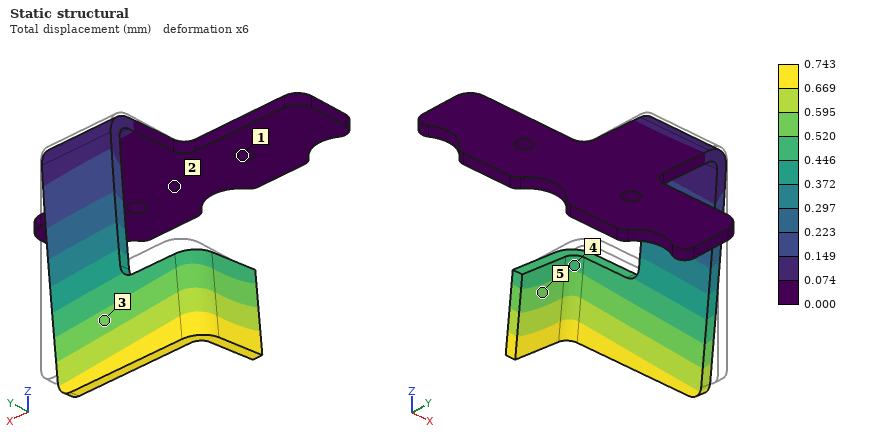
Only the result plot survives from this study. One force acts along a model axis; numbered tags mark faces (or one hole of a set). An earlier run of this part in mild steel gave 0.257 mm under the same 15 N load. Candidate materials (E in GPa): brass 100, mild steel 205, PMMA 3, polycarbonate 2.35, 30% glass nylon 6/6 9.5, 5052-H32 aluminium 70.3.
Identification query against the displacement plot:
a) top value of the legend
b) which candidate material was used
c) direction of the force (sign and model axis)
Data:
0.743 mm
5052-H32 aluminium
-Y
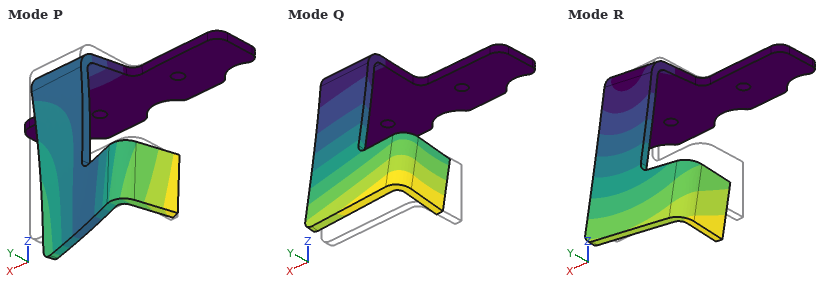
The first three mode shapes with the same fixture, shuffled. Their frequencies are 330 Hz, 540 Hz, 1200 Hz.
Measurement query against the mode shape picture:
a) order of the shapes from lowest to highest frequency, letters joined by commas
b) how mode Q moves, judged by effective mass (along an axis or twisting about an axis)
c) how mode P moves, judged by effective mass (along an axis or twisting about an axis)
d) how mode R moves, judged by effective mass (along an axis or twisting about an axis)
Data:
Q, R, P
along Y
along Z
along X
